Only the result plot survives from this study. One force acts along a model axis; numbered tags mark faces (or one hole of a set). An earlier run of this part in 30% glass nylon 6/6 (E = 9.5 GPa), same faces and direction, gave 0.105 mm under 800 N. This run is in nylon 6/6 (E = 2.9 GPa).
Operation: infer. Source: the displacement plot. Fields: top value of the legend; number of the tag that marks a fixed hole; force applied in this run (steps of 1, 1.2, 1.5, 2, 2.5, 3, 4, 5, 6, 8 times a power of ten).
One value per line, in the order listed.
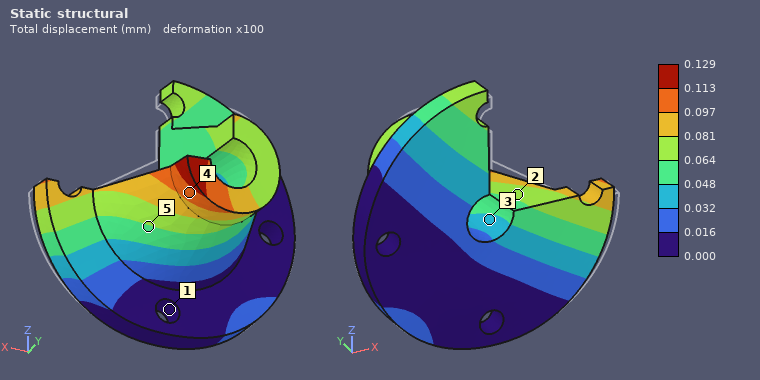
0.129 mm
1
300 N
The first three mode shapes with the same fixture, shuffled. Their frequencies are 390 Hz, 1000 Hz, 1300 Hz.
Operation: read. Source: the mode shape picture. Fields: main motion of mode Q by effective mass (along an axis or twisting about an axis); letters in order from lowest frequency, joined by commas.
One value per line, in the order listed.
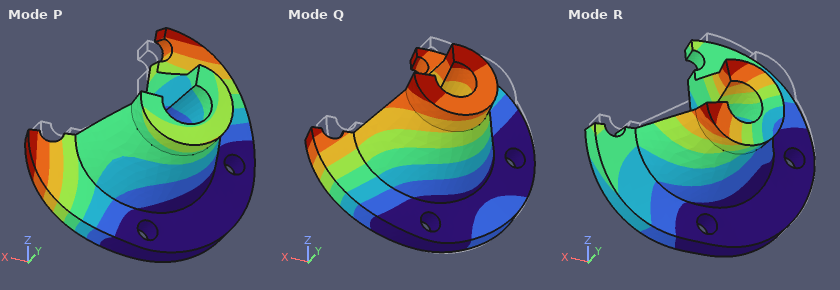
along Y
Q, P, R
